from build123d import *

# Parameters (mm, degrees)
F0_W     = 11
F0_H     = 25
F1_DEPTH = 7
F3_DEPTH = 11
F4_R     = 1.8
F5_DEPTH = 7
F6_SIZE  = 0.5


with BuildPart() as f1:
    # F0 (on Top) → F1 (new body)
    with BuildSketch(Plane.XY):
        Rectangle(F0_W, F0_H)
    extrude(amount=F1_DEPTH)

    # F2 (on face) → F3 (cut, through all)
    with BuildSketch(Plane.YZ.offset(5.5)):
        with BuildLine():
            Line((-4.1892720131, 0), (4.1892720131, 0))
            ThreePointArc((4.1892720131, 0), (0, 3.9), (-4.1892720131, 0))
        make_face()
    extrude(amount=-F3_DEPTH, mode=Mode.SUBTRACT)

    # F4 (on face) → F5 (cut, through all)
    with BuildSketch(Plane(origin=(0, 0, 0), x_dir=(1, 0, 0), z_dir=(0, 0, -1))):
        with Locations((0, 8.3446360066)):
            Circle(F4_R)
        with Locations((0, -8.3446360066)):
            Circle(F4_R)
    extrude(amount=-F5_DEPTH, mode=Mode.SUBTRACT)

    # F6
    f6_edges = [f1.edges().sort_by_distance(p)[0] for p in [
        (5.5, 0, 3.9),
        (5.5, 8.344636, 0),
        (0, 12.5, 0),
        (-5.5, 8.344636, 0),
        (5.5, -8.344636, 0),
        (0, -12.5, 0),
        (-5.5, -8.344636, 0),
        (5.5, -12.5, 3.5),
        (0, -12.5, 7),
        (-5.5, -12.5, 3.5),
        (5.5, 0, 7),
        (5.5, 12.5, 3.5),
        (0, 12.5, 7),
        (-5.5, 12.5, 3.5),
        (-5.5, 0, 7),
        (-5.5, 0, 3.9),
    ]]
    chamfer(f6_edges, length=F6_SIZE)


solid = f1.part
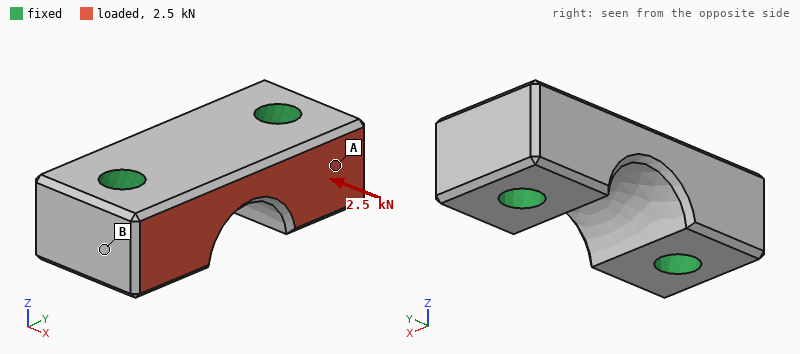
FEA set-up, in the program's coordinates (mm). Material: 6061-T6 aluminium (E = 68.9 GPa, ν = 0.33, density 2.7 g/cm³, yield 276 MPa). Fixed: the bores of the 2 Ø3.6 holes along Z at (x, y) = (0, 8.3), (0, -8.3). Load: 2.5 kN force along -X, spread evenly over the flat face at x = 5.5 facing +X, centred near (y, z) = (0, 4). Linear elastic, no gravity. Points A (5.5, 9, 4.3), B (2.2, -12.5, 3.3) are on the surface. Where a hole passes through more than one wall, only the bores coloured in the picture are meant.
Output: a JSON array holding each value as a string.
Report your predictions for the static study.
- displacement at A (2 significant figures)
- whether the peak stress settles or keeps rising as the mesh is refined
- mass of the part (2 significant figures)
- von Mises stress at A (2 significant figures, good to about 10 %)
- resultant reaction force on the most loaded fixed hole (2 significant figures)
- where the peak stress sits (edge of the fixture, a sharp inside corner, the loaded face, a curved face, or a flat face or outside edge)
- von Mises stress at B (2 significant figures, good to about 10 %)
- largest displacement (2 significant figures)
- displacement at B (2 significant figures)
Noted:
["1.3 µm", "keeps rising", "4.0 g", "22 MPa", "1.3 kN", "edge of the fixture", "9.5 MPa", "3.2 µm", "0.60 µm"]
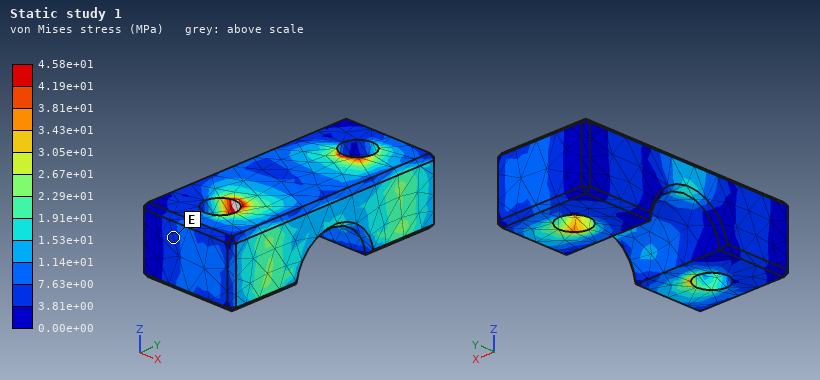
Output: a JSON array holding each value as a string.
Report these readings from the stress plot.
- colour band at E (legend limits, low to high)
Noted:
["3.81e+00 to 7.63e+00 MPa"]
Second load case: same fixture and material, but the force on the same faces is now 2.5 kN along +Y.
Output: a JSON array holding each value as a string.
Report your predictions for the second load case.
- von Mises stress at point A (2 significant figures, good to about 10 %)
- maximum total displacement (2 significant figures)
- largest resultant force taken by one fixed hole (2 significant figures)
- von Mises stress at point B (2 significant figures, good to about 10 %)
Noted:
["41 MPa", "6.6 µm", "1.3 kN", "35 MPa"]
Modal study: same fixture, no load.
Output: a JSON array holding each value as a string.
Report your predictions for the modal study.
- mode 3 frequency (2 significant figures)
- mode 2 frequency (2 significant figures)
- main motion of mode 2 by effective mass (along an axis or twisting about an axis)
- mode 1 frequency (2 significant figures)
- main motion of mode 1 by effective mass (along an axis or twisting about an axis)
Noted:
["100 kHz", "87 kHz", "along Z", "79 kHz", "along X"]
